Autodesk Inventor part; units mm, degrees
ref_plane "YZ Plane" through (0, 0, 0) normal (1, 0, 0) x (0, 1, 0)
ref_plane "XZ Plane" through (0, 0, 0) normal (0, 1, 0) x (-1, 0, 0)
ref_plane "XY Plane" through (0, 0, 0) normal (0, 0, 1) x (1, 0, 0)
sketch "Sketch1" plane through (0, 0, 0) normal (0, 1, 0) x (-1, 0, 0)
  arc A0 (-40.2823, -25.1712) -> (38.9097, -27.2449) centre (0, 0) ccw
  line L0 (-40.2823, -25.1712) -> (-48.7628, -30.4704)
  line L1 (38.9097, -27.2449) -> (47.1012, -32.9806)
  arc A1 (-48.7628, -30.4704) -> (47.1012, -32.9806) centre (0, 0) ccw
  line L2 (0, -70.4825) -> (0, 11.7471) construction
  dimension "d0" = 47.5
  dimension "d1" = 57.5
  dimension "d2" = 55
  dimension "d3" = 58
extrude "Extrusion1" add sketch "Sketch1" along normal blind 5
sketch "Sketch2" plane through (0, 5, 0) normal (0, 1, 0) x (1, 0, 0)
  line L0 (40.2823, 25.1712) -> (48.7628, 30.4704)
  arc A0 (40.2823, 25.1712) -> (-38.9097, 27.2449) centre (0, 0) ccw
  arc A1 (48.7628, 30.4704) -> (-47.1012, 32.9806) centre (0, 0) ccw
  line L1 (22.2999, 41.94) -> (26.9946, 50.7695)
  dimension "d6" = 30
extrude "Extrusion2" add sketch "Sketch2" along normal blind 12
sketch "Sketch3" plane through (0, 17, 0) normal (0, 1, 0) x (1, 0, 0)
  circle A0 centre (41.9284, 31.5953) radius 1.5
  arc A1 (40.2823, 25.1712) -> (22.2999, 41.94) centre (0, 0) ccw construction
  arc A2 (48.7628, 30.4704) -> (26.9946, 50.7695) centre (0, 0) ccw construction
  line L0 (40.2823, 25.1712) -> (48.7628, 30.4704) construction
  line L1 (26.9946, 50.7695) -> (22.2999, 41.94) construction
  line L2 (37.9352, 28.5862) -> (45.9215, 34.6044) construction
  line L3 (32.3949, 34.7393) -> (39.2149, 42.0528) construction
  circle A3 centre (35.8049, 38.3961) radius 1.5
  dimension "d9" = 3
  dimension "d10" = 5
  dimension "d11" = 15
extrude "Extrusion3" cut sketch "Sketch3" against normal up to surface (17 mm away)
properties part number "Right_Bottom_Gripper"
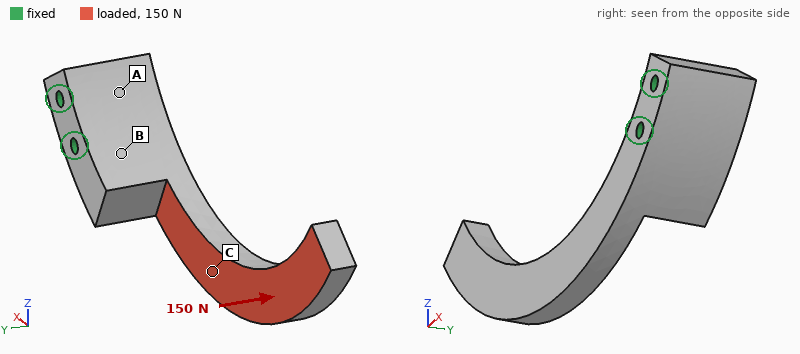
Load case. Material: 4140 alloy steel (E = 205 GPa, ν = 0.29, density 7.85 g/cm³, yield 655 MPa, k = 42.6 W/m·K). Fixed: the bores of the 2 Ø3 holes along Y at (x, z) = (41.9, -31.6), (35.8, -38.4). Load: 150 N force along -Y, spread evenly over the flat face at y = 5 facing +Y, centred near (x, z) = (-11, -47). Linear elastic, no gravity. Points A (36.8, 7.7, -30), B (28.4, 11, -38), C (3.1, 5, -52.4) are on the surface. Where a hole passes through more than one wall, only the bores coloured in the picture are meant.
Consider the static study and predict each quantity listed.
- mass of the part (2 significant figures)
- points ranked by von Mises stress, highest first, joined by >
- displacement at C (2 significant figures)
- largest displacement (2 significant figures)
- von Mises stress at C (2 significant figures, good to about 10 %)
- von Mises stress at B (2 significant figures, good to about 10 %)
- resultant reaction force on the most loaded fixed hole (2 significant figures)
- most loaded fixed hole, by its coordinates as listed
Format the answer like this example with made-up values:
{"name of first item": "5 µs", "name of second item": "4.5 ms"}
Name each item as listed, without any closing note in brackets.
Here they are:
{"mass of the part": "65 g", "points ranked by von Mises stress, highest first, joined by >": "C > B > A", "displacement at C": "0.070 mm", "largest displacement": "0.41 mm", "von Mises stress at C": "64 MPa", "von Mises stress at B": "18 MPa", "resultant reaction force on the most loaded fixed hole": "190 N", "most loaded fixed hole, by its coordinates as listed": "(35.8, -38.4)"}
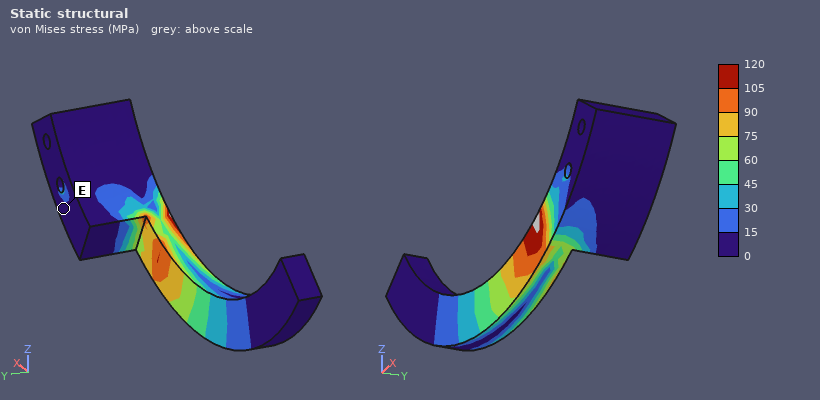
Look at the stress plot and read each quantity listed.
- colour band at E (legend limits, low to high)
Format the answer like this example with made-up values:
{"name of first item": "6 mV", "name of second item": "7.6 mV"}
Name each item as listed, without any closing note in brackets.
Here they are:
{"colour band at E": "0 to 15 MPa"}
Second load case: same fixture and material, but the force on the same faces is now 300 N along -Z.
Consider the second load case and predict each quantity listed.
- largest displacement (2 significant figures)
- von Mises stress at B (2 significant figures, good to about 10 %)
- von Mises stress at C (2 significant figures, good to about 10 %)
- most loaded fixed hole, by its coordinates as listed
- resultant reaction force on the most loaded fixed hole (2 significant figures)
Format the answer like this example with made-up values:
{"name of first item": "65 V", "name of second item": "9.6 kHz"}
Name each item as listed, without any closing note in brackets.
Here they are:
{"largest displacement": "0.28 mm", "von Mises stress at B": "38 MPa", "von Mises stress at C": "25 MPa", "most loaded fixed hole, by its coordinates as listed": "(35.8, -38.4)", "resultant reaction force on the most loaded fixed hole": "990 N"}
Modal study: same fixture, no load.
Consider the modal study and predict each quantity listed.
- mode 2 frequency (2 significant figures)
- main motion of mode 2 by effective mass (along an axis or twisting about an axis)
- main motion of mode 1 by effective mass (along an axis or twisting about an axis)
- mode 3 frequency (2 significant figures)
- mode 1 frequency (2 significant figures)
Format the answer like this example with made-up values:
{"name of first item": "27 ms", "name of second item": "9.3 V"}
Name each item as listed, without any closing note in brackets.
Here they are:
{"mode 2 frequency": "1200 Hz", "main motion of mode 2 by effective mass": "along Z", "main motion of mode 1 by effective mass": "along Y", "mode 3 frequency": "3300 Hz", "mode 1 frequency": "700 Hz"}
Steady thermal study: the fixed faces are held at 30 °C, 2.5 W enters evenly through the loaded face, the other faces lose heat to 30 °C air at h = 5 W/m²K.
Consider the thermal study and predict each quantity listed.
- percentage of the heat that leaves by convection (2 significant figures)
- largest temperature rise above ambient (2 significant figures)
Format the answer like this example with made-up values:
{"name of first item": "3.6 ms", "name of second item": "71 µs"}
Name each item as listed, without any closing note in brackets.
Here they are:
{"percentage of the heat that leaves by convection": "11 %", "largest temperature rise above ambient": "46 K"}
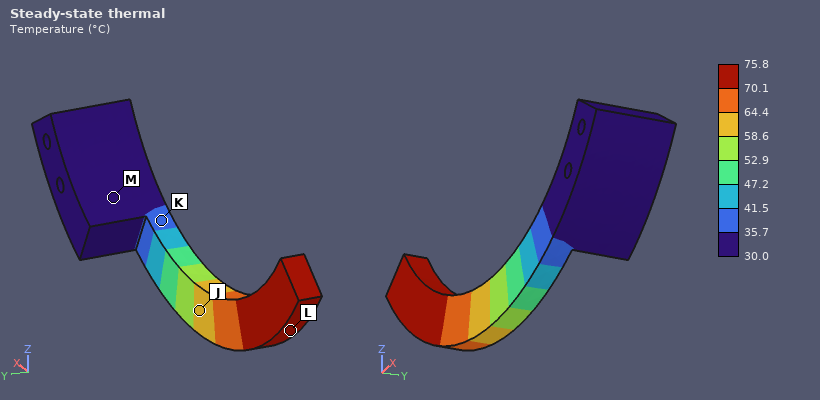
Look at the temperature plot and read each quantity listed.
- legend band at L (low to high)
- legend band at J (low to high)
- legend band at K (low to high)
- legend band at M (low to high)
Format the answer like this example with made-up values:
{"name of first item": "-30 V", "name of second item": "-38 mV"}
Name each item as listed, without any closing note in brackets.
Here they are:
{"legend band at L": "70.1 to 75.8 °C", "legend band at J": "58.6 to 64.4 °C", "legend band at K": "35.7 to 41.5 °C", "legend band at M": "30.0 to 35.7 °C"}
